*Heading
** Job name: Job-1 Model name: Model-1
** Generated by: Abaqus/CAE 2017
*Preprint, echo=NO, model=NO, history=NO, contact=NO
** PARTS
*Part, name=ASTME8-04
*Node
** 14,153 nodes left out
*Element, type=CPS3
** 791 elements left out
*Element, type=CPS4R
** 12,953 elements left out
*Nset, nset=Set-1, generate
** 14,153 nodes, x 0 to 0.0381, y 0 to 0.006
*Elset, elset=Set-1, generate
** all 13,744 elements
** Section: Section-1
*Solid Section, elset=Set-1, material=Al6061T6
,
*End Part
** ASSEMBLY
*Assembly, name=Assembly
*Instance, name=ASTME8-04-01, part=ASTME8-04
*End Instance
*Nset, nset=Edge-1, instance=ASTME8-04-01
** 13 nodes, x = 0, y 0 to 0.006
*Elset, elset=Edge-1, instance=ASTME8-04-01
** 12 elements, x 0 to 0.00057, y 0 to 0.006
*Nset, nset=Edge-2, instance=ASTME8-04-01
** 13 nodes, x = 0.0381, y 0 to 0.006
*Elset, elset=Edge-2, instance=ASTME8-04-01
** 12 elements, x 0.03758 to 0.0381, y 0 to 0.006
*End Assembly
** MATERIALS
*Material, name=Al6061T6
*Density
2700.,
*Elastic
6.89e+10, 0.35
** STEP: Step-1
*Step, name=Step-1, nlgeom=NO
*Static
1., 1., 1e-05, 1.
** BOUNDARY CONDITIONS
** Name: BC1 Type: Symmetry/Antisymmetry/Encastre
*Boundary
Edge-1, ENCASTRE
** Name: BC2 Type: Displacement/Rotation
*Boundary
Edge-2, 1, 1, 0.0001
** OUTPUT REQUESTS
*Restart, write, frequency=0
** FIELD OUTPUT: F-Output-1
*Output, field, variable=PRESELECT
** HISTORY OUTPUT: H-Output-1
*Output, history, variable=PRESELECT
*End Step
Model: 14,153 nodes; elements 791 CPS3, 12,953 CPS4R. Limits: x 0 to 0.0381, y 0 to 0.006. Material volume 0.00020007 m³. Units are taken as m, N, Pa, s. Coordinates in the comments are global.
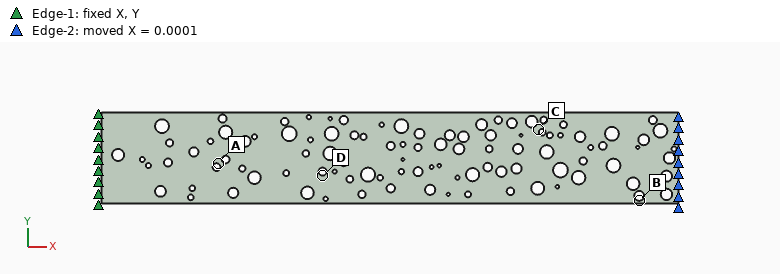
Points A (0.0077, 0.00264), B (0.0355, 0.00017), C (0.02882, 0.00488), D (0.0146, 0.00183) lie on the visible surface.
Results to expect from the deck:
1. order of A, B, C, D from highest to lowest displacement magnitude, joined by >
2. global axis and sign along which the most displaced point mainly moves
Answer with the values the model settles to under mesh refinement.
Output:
B > C > D > A
+X
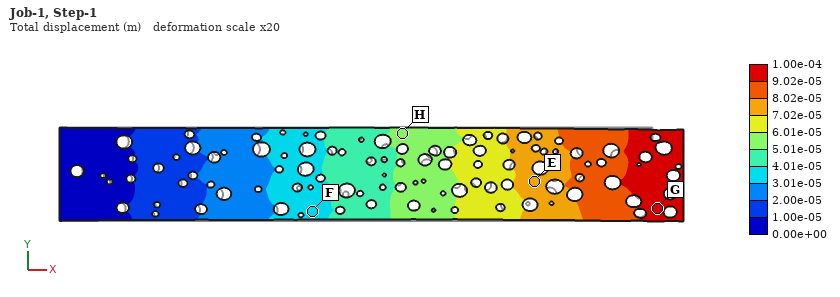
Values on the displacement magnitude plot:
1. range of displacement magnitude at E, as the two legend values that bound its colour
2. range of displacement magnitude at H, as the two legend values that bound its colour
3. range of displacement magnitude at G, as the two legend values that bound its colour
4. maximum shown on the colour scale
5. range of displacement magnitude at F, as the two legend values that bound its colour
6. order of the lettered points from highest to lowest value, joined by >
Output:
7.02e-05 to 8.02e-05 m
5.01e-05 to 6.01e-05 m
9.02e-05 to 1.00e-04 m
1.00e-04 m
3.01e-05 to 4.01e-05 m
G > E > H > F
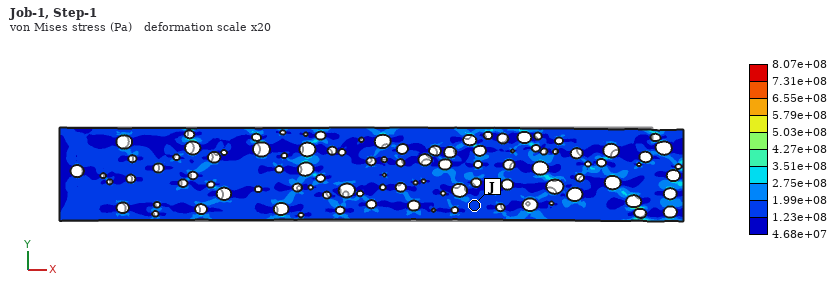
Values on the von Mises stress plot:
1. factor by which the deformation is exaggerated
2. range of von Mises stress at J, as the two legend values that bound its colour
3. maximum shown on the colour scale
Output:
20
1.23e+08 to 1.99e+08 Pa
8.07e+08 Pa
